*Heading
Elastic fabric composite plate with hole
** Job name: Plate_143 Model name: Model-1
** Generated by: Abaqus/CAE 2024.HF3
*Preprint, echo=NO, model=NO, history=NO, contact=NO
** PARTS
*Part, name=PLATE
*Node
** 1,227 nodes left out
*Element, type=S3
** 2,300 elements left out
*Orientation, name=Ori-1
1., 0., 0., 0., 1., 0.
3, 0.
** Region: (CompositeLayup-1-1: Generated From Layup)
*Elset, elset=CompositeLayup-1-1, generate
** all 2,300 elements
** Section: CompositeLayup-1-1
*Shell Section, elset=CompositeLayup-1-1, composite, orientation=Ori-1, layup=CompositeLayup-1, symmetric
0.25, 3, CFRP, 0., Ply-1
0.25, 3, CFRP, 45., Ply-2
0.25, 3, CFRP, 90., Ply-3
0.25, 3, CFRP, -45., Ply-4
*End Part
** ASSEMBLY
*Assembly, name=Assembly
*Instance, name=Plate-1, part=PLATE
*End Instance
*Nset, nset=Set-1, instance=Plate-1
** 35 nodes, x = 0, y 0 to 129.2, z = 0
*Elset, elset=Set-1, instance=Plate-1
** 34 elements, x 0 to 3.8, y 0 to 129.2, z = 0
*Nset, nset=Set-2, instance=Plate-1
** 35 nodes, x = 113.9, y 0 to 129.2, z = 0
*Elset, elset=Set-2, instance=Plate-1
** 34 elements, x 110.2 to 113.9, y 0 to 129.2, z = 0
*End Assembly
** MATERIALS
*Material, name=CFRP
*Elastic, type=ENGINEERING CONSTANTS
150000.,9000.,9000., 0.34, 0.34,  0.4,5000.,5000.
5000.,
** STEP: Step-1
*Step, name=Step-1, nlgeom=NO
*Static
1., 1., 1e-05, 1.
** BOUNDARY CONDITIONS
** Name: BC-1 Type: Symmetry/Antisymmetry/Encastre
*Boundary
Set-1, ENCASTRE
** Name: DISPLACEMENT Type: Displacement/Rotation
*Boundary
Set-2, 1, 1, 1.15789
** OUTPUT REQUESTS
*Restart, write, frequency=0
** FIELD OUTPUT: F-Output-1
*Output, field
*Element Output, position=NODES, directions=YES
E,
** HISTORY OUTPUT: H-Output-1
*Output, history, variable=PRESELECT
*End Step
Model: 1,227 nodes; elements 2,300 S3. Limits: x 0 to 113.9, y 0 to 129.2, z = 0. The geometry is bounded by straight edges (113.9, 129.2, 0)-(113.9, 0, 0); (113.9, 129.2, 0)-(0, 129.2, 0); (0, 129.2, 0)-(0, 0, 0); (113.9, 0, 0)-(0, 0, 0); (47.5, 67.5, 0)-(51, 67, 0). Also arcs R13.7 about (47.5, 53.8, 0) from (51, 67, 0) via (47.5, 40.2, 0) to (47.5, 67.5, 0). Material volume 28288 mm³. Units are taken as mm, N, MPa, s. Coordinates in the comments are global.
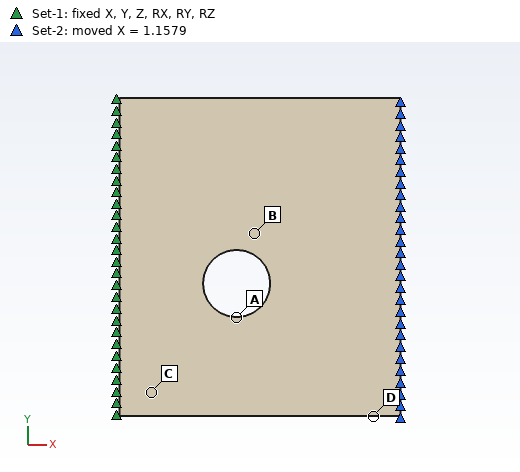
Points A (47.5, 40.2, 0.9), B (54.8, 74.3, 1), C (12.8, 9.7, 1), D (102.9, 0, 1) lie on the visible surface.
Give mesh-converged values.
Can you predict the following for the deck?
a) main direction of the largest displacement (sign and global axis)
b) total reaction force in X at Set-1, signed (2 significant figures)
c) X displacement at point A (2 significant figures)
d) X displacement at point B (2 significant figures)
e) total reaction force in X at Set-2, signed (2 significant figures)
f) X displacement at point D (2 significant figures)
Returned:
+X
-1.4e+05 N
0.48 mm
0.57 mm
1.4e+05 N
1.0 mm
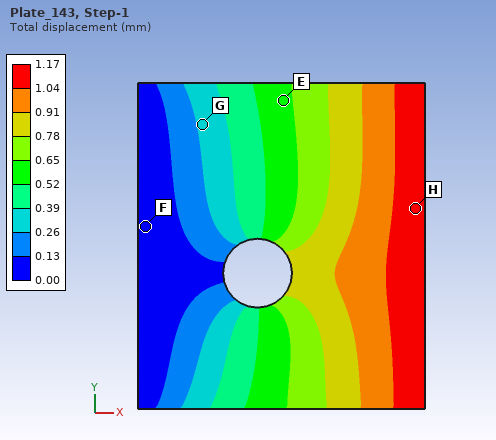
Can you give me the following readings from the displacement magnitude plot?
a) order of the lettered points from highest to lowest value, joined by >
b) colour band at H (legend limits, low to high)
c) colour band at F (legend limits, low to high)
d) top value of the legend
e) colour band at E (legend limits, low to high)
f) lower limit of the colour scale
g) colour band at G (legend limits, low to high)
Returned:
H > E > G > F
1.04 to 1.17 mm
0.00 to 0.13 mm
1.17 mm
0.52 to 0.65 mm
0.00 mm
0.26 to 0.39 mm
